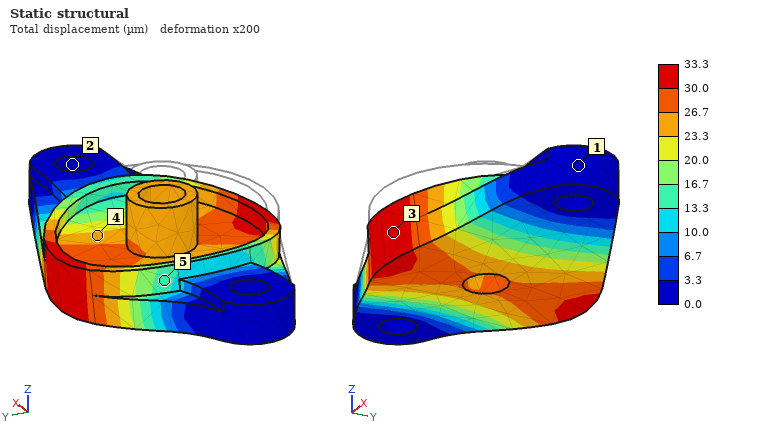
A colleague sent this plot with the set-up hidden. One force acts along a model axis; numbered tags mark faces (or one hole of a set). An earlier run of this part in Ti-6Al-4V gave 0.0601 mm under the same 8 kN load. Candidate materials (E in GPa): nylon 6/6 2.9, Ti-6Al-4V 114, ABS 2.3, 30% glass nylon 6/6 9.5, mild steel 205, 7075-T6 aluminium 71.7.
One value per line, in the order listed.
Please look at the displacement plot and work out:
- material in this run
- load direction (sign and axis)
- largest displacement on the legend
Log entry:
mild steel
-Z
33.3 µm
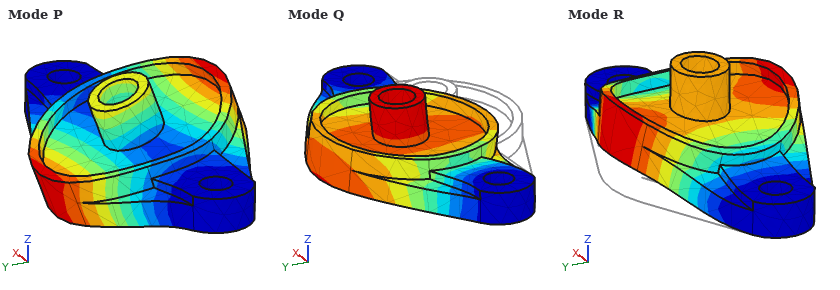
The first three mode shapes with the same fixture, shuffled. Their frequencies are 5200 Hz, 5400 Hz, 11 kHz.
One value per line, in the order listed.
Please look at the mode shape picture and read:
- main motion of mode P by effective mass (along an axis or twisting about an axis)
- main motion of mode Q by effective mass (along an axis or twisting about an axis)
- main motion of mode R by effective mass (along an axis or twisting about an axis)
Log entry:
twisting about X
along Y
along Z
